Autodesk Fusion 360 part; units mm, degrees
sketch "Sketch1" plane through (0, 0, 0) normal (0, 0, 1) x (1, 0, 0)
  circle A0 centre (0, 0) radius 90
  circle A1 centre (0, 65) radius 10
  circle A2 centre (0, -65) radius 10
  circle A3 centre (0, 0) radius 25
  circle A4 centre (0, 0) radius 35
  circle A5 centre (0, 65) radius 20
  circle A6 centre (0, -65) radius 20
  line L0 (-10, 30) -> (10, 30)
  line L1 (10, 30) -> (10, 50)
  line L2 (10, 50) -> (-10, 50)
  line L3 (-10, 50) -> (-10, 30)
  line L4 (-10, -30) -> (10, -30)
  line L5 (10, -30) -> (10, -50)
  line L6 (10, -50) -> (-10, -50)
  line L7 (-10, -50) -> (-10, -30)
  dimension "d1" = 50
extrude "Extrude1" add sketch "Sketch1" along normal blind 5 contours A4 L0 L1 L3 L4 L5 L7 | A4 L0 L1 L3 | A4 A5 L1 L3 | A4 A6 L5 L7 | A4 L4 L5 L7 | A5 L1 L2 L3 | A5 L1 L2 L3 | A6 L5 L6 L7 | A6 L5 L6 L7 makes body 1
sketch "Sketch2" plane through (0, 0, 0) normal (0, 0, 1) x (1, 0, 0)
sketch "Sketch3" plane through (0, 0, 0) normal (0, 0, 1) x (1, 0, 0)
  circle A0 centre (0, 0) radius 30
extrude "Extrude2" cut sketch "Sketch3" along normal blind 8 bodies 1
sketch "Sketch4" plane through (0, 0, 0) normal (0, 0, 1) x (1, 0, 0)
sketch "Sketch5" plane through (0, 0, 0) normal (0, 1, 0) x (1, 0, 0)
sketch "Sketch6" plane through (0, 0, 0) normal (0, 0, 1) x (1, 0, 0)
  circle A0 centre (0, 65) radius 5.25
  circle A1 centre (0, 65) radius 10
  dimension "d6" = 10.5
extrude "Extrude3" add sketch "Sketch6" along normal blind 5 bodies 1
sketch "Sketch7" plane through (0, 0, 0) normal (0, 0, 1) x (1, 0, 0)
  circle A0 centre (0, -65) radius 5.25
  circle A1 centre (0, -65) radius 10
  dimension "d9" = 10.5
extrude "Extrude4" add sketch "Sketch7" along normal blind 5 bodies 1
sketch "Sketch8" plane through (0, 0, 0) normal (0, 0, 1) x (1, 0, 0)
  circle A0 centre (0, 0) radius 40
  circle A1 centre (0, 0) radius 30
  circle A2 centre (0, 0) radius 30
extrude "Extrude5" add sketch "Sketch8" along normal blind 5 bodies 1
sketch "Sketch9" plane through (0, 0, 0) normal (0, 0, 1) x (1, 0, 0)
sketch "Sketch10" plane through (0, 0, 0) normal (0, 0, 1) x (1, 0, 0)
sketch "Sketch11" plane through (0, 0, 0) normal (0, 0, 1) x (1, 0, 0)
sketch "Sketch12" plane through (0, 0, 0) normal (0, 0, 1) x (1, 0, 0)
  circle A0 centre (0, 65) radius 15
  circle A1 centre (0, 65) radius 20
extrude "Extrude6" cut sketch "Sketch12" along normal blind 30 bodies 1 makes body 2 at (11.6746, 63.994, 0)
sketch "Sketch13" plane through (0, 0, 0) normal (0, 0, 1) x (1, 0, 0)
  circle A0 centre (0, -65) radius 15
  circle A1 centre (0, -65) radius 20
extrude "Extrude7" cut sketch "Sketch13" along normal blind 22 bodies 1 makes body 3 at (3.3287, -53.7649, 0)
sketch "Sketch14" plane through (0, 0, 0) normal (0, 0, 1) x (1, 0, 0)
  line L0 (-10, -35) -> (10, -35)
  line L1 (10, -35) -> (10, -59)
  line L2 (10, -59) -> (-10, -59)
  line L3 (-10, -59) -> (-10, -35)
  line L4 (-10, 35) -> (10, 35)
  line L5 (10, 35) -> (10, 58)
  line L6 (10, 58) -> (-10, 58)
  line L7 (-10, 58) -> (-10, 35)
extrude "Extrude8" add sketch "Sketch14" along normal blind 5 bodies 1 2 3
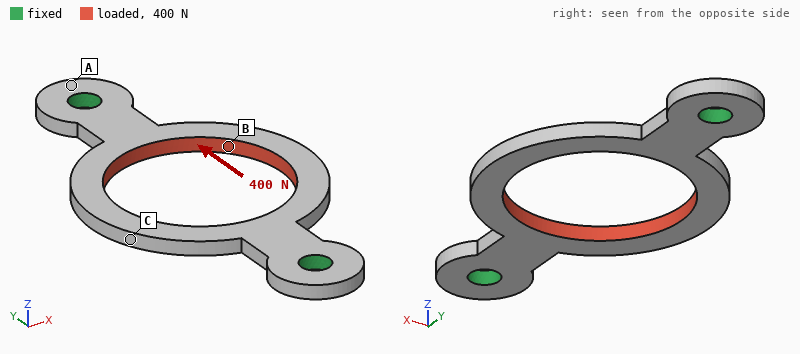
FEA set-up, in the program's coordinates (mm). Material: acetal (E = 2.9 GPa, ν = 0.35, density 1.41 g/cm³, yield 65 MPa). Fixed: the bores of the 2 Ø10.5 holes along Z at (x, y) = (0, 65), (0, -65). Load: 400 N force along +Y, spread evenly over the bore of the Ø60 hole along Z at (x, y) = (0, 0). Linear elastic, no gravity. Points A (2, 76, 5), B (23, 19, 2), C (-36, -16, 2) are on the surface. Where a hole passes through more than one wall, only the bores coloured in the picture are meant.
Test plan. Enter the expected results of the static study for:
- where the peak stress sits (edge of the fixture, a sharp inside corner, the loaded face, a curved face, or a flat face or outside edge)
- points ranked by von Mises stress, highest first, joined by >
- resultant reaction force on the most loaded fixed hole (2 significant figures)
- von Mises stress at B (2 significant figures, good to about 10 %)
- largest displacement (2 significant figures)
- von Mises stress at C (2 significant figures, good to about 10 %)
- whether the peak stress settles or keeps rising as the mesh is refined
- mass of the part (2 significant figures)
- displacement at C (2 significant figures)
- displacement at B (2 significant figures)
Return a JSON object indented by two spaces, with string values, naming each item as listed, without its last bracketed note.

{
  "where the peak stress sits": "a sharp inside corner",
  "points ranked by von Mises stress, highest first, joined by >": "B > C > A",
  "resultant reaction force on the most loaded fixed hole": "200 N",
  "von Mises stress at B": "5.8 MPa",
  "largest displacement": "0.12 mm",
  "von Mises stress at C": "3.0 MPa",
  "whether the peak stress settles or keeps rising as the mesh is refined": "keeps rising",
  "mass of the part": "28 g",
  "displacement at C": "0.11 mm",
  "displacement at B": "0.11 mm"
}
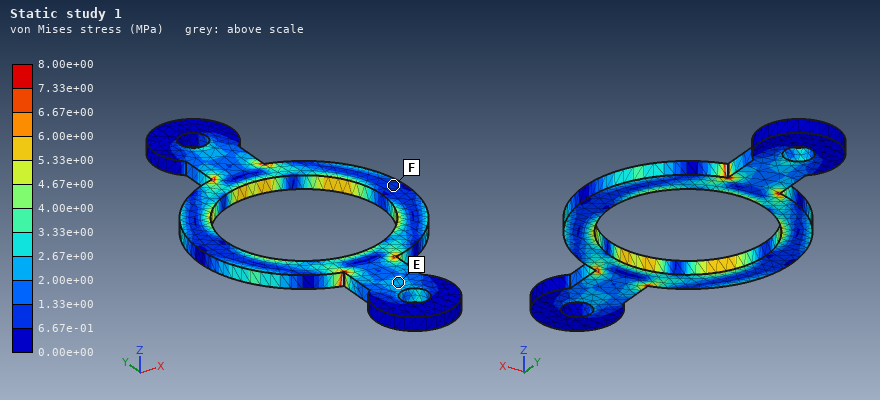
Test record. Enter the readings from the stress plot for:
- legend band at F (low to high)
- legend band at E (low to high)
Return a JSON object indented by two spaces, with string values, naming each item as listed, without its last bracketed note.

{
  "legend band at F": "6.67e-01 to 1.33e+00 MPa",
  "legend band at E": "2.00e+00 to 2.67e+00 MPa"
}
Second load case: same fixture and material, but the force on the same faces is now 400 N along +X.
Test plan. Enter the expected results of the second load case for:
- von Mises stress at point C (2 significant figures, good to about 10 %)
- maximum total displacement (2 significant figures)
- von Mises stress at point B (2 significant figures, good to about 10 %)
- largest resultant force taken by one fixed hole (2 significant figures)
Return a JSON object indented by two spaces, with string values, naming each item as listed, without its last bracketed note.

{
  "von Mises stress at point C": "0.91 MPa",
  "maximum total displacement": "0.15 mm",
  "von Mises stress at point B": "2.2 MPa",
  "largest resultant force taken by one fixed hole": "200 N"
}
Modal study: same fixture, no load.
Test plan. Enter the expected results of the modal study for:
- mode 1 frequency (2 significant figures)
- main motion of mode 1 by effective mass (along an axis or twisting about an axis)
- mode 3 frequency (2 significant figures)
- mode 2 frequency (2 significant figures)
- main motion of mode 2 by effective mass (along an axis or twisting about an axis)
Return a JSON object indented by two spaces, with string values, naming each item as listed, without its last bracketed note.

{
  "mode 1 frequency": "340 Hz",
  "main motion of mode 1 by effective mass": "twisting about Y",
  "mode 3 frequency": "970 Hz",
  "mode 2 frequency": "380 Hz",
  "main motion of mode 2 by effective mass": "along Z"
}
